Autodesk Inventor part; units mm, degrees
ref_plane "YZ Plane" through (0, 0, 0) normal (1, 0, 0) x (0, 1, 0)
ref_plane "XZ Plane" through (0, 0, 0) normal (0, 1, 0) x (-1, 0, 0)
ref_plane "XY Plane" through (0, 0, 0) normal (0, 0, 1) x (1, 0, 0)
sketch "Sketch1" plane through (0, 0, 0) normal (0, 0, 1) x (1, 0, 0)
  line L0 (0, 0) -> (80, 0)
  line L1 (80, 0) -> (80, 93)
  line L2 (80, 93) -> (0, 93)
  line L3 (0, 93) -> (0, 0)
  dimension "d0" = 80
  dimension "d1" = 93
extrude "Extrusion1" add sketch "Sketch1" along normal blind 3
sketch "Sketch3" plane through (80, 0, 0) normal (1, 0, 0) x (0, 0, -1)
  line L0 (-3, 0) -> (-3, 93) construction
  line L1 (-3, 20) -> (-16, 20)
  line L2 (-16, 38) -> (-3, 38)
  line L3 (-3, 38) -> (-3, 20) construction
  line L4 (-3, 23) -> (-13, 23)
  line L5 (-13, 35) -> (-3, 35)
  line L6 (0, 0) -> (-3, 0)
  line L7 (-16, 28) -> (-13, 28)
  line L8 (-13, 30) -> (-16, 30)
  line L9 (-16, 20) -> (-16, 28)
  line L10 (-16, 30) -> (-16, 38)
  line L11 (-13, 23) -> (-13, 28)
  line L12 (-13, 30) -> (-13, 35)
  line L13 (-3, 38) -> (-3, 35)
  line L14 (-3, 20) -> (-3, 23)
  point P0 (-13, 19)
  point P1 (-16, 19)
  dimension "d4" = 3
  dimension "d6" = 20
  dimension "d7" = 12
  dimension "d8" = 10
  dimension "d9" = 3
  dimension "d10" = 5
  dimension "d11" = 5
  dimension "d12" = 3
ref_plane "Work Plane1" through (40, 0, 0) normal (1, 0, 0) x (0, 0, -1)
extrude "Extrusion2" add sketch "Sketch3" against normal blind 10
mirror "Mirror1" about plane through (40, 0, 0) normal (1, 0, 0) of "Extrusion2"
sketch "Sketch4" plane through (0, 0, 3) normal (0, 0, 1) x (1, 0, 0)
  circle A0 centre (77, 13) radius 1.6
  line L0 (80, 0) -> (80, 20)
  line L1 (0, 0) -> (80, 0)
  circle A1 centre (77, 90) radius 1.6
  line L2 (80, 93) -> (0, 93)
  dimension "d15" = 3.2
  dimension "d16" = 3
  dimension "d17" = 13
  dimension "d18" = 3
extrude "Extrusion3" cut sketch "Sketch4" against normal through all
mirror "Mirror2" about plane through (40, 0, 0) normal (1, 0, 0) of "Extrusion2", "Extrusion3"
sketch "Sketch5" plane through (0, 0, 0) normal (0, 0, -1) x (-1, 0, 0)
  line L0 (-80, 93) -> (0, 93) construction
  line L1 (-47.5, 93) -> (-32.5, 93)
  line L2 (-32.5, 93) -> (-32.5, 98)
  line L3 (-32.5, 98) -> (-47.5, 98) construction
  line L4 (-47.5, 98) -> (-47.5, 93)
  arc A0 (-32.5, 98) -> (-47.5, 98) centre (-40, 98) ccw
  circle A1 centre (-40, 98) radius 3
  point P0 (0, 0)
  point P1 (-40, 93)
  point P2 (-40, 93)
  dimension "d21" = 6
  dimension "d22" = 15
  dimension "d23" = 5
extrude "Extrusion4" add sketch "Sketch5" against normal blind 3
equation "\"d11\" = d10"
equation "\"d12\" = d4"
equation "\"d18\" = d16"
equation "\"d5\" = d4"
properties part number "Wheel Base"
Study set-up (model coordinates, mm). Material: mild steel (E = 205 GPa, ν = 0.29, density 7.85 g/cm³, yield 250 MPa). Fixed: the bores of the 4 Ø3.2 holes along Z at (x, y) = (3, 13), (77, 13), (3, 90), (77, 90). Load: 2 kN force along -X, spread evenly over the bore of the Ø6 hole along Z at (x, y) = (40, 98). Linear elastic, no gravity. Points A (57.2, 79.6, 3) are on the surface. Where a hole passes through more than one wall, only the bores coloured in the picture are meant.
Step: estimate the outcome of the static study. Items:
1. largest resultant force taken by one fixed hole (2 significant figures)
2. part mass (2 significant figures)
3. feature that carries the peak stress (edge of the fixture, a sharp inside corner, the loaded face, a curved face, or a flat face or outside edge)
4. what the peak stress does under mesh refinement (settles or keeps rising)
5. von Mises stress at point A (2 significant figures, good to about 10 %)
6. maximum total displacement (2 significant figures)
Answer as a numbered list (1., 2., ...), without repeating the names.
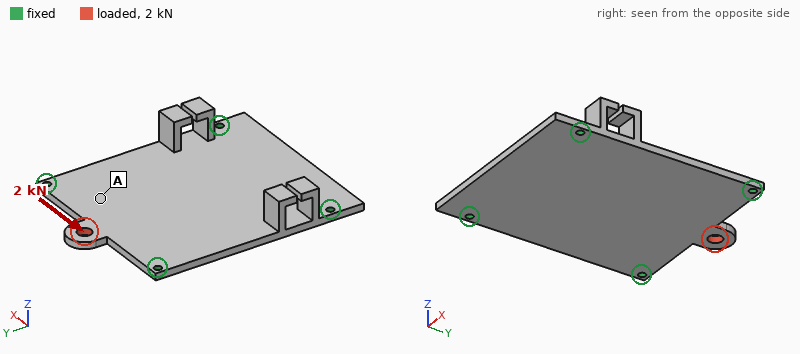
1. 890 N
2. 190 g
3. a sharp inside corner
4. keeps rising
5. 14 MPa
6. 23 µm
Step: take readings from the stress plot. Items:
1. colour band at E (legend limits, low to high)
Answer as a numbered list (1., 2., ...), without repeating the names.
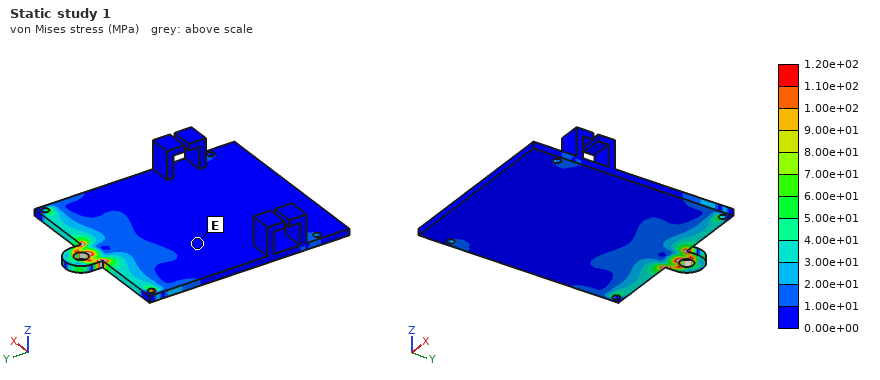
1. 0.00e+00 to 1.00e+01 MPa
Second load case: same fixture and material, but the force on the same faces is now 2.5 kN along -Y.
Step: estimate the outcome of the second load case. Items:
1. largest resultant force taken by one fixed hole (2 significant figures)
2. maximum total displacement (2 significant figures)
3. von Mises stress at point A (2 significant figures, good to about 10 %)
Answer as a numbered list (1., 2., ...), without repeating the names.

1. 680 N
2. 11 µm
3. 17 MPa
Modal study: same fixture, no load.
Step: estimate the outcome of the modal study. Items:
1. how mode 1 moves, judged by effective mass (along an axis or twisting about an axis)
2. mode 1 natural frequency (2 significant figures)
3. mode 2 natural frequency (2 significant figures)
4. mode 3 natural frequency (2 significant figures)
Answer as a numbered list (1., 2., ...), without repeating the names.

1. along Z
2. 1600 Hz
3. 2600 Hz
4. 2700 Hz
